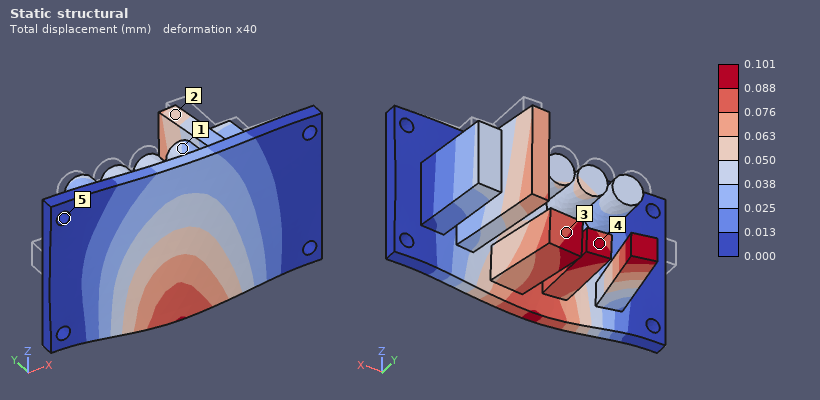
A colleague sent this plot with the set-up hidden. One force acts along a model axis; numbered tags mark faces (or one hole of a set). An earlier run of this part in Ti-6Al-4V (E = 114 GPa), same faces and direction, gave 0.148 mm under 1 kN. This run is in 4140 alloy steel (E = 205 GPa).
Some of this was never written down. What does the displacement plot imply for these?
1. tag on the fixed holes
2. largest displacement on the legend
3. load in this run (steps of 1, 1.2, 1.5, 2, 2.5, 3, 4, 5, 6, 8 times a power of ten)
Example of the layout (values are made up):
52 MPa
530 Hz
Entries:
5
0.101 mm
1.2 kN
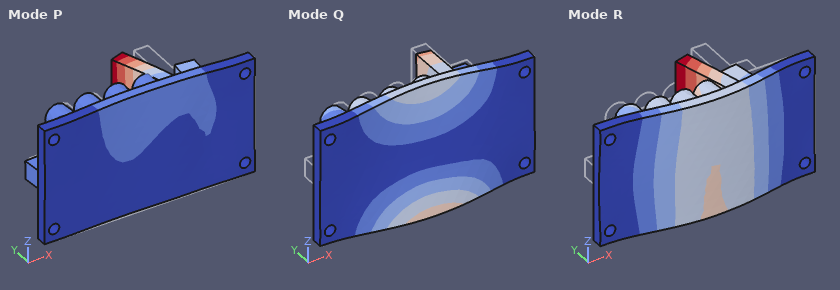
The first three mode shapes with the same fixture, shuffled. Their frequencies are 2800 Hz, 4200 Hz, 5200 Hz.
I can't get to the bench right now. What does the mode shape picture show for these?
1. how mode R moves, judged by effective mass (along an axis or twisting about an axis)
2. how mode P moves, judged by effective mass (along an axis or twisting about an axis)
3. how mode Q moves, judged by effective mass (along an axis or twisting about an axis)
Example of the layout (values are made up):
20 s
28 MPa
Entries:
along Y
along Y
along Z
